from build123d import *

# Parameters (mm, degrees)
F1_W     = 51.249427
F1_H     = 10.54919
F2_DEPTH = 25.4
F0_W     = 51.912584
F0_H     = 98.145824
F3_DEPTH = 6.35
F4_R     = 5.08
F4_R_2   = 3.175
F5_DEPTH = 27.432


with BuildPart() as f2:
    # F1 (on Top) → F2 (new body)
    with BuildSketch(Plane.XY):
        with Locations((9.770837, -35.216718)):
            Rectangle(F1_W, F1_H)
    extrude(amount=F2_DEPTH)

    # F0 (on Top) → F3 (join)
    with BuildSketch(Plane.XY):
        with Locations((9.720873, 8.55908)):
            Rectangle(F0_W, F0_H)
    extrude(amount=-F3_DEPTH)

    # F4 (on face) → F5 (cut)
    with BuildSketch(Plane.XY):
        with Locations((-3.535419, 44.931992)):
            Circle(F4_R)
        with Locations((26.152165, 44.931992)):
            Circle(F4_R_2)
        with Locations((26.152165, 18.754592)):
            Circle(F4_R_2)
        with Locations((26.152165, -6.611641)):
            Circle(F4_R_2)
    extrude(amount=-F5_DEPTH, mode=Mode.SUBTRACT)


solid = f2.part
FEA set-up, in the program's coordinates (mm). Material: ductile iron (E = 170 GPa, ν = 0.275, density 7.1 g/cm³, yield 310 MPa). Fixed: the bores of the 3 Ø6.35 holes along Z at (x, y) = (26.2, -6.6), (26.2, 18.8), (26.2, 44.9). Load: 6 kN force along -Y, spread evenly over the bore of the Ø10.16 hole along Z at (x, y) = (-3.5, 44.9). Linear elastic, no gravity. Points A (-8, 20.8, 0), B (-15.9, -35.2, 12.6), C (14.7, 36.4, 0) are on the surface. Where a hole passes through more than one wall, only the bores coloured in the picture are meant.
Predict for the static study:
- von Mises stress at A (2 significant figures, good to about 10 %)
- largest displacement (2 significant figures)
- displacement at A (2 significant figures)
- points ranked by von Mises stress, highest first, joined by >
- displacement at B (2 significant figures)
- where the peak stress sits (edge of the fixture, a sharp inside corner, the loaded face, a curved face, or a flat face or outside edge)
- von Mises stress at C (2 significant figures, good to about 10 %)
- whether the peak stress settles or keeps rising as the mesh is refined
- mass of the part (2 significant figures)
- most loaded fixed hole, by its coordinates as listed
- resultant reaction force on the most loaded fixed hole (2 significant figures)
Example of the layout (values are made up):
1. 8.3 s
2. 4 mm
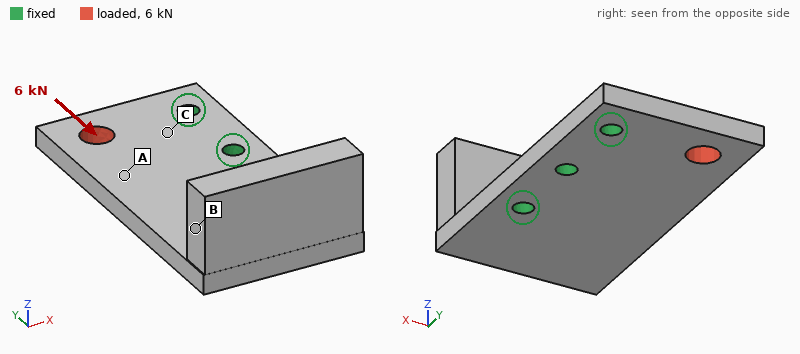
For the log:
1. 23 MPa
2. 15 µm
3. 8.5 µm
4. C > A > B
5. 10 µm
6. edge of the fixture
7. 38 MPa
8. keeps rising
9. 320 g
10. (26.2, 44.9)
11. 3.9 kN
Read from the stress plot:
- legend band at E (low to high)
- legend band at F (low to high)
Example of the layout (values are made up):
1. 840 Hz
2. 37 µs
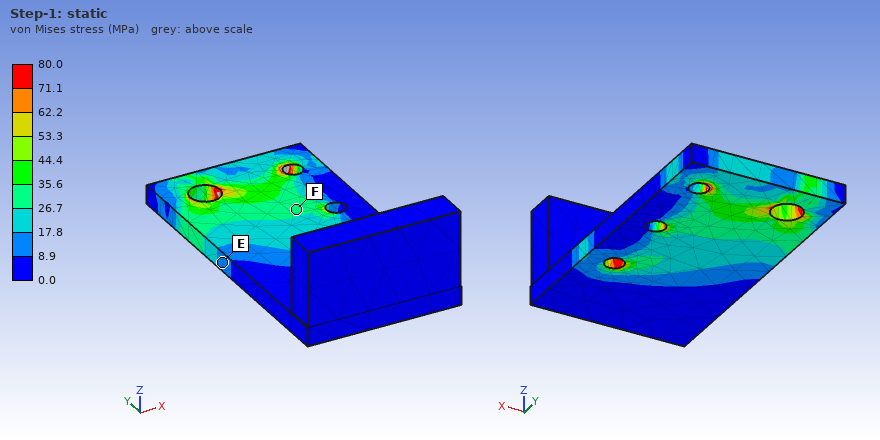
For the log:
1. 8.9 to 17.8 MPa
2. 26.7 to 35.6 MPa
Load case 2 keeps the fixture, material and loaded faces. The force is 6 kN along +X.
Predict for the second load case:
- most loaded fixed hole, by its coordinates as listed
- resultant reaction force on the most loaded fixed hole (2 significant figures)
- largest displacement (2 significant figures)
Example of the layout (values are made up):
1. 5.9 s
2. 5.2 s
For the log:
1. (26.2, 44.9)
2. 5.1 kN
3. 11 µm
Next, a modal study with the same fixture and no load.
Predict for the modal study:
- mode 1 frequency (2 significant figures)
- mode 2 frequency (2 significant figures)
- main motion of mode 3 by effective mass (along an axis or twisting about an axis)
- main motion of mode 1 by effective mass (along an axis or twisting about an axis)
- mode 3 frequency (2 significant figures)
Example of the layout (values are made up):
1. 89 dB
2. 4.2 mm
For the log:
1. 1300 Hz
2. 2100 Hz
3. along Z
4. along Z
5. 3600 Hz
